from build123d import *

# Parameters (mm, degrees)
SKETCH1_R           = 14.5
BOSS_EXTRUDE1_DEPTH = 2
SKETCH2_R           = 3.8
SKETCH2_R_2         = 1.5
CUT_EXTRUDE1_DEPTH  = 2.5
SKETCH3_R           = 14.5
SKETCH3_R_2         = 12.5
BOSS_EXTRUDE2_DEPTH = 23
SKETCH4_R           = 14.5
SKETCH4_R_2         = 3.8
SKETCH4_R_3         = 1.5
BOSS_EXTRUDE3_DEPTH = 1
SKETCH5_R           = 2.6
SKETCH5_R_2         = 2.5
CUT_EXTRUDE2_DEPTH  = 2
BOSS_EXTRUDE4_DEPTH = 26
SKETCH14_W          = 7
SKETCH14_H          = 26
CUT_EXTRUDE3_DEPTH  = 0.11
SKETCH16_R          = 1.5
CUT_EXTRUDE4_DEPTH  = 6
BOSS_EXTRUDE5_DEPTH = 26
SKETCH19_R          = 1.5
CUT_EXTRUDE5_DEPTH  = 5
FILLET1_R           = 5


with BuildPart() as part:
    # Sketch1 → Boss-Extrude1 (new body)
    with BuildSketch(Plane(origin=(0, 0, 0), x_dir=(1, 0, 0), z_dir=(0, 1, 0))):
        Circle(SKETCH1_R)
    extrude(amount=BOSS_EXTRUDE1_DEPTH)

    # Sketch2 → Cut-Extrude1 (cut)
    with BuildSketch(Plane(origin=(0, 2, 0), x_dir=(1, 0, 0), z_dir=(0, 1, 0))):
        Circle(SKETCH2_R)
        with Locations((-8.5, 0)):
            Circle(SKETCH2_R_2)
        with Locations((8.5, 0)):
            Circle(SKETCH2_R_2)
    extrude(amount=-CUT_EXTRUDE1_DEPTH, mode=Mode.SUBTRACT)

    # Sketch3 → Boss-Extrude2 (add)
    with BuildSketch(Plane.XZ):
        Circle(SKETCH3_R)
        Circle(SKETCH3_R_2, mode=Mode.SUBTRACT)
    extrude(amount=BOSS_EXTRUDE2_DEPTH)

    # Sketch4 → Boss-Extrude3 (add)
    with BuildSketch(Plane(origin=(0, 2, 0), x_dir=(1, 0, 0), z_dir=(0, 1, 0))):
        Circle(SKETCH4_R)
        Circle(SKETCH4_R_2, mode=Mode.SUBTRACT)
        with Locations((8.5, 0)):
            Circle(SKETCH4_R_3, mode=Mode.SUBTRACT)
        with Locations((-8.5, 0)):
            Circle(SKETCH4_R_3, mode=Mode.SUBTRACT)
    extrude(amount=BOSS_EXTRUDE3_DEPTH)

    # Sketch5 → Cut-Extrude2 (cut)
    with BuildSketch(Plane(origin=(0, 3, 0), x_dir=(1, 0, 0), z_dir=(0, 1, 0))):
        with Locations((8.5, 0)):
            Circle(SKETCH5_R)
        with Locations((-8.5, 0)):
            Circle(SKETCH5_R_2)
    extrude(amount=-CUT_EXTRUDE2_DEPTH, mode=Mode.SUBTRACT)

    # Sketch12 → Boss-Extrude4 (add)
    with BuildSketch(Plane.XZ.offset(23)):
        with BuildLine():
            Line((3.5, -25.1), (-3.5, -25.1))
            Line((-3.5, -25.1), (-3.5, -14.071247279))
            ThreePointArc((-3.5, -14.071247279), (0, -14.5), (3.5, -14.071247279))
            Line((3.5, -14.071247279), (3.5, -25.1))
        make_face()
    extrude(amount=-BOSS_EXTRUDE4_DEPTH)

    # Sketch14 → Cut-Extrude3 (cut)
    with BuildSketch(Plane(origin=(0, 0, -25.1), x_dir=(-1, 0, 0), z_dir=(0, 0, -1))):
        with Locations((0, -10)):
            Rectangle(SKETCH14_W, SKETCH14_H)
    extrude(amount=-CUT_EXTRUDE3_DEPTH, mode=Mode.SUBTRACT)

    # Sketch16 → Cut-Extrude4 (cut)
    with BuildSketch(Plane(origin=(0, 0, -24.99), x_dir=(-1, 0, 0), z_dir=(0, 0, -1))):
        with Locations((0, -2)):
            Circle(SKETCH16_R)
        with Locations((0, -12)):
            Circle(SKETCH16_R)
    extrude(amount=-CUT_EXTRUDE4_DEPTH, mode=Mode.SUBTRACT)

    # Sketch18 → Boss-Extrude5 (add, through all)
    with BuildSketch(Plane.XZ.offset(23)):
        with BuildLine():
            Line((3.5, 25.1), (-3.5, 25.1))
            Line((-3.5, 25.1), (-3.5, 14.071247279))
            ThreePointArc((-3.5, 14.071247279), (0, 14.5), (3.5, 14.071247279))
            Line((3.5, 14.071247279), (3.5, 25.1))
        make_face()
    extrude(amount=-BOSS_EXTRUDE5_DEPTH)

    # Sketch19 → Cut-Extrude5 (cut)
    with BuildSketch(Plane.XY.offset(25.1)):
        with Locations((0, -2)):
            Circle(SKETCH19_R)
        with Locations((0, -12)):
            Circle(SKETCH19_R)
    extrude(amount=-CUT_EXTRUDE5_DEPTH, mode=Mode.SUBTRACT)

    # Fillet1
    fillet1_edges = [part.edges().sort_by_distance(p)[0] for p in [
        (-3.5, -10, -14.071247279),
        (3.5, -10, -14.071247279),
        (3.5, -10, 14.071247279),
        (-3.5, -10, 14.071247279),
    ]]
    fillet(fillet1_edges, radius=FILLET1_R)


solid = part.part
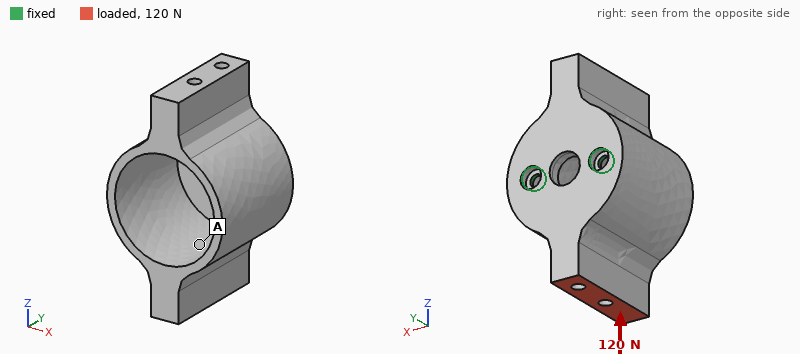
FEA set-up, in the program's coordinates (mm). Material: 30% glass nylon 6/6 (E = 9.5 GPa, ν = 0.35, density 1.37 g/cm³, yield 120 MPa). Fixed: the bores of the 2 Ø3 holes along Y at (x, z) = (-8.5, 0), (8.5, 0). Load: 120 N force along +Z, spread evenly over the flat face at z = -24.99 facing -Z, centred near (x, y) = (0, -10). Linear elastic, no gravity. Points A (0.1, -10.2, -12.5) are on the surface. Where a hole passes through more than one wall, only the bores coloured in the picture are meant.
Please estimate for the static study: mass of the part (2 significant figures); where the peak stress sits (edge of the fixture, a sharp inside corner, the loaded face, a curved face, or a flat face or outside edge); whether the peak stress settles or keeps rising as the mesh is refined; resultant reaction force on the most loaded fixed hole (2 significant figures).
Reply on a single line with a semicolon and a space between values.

13 g; edge of the fixture; keeps rising; 63 N
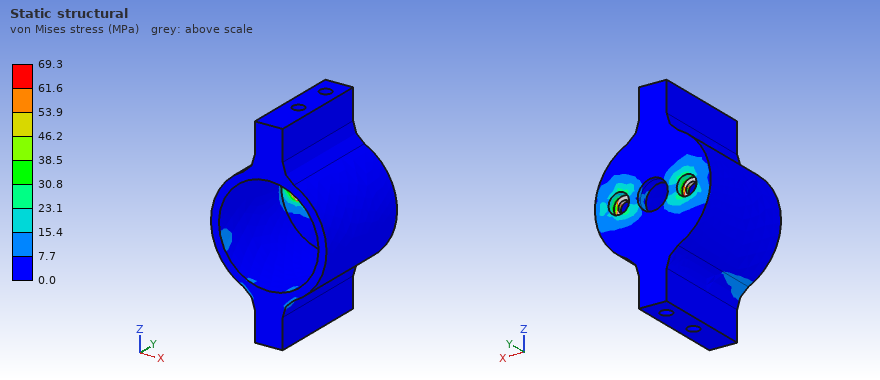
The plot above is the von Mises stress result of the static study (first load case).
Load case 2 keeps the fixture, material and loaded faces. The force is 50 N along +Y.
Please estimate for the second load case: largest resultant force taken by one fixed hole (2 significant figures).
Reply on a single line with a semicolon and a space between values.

25 N
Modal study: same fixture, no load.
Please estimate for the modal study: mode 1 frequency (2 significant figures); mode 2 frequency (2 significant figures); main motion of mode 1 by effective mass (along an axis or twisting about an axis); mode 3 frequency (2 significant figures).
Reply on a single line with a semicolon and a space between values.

610 Hz; 2800 Hz; along Z; 2900 Hz
